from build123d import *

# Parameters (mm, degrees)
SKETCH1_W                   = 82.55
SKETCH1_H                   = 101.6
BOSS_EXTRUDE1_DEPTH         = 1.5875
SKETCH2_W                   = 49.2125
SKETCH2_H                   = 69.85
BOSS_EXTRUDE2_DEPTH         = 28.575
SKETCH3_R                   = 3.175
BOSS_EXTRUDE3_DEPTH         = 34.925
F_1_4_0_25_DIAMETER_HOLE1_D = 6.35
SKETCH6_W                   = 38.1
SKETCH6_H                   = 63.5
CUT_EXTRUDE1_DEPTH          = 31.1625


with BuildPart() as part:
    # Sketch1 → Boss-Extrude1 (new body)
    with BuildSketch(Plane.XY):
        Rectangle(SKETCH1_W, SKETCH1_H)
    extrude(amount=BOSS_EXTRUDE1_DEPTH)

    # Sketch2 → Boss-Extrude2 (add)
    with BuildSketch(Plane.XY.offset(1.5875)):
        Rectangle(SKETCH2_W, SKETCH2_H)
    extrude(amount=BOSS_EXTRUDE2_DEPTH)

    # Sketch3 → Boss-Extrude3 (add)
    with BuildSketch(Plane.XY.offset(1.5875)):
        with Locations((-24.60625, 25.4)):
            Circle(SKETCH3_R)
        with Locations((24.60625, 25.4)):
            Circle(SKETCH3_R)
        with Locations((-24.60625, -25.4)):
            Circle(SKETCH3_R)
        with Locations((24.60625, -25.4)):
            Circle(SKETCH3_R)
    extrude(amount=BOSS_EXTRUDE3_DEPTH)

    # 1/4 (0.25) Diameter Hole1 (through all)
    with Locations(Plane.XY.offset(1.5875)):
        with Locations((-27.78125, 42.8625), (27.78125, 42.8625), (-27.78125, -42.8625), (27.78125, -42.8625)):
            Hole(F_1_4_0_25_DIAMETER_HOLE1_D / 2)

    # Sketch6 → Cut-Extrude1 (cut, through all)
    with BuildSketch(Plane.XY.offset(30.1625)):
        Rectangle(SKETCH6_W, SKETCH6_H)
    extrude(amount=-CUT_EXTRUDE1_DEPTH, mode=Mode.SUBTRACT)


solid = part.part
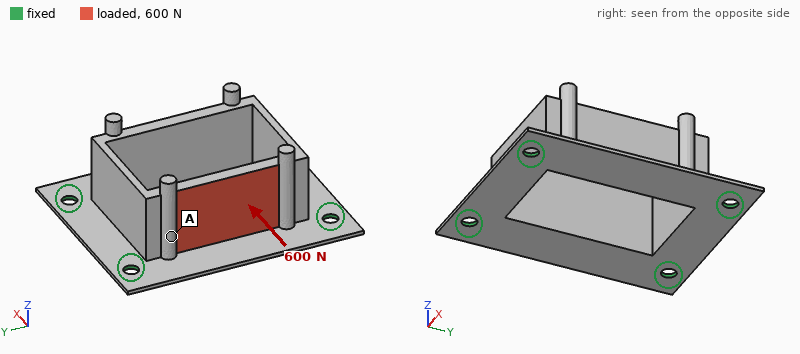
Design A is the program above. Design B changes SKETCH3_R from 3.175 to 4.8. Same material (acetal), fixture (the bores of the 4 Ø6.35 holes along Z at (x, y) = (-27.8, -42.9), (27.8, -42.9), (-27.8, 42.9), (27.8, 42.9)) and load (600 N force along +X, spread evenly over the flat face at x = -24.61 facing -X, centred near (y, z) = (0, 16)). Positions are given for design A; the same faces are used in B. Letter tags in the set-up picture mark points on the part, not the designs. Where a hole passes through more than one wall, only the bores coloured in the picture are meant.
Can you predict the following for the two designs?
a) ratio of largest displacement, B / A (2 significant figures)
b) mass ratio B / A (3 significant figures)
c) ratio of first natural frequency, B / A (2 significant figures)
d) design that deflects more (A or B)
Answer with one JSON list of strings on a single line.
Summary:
["0.90", "1.08", "0.96", "A"]
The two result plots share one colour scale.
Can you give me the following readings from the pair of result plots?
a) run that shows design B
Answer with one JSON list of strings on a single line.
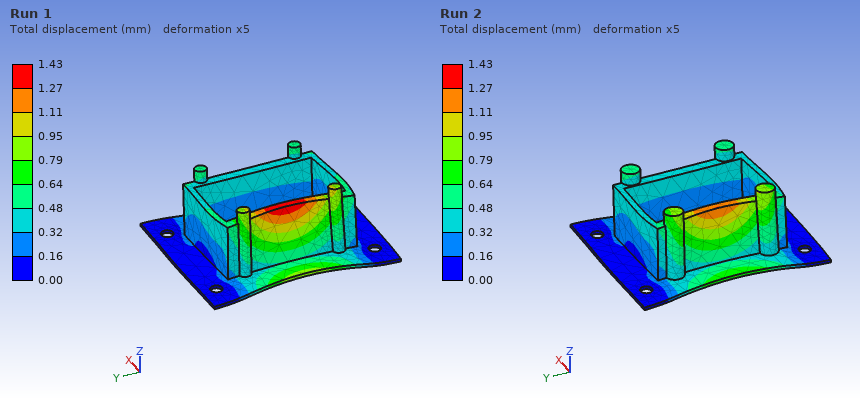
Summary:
["Run 2"]
